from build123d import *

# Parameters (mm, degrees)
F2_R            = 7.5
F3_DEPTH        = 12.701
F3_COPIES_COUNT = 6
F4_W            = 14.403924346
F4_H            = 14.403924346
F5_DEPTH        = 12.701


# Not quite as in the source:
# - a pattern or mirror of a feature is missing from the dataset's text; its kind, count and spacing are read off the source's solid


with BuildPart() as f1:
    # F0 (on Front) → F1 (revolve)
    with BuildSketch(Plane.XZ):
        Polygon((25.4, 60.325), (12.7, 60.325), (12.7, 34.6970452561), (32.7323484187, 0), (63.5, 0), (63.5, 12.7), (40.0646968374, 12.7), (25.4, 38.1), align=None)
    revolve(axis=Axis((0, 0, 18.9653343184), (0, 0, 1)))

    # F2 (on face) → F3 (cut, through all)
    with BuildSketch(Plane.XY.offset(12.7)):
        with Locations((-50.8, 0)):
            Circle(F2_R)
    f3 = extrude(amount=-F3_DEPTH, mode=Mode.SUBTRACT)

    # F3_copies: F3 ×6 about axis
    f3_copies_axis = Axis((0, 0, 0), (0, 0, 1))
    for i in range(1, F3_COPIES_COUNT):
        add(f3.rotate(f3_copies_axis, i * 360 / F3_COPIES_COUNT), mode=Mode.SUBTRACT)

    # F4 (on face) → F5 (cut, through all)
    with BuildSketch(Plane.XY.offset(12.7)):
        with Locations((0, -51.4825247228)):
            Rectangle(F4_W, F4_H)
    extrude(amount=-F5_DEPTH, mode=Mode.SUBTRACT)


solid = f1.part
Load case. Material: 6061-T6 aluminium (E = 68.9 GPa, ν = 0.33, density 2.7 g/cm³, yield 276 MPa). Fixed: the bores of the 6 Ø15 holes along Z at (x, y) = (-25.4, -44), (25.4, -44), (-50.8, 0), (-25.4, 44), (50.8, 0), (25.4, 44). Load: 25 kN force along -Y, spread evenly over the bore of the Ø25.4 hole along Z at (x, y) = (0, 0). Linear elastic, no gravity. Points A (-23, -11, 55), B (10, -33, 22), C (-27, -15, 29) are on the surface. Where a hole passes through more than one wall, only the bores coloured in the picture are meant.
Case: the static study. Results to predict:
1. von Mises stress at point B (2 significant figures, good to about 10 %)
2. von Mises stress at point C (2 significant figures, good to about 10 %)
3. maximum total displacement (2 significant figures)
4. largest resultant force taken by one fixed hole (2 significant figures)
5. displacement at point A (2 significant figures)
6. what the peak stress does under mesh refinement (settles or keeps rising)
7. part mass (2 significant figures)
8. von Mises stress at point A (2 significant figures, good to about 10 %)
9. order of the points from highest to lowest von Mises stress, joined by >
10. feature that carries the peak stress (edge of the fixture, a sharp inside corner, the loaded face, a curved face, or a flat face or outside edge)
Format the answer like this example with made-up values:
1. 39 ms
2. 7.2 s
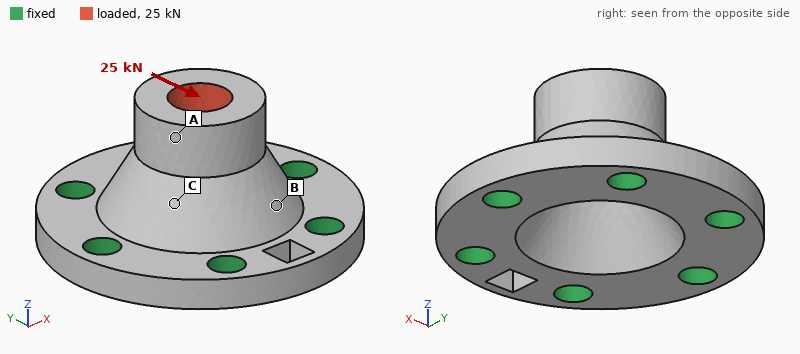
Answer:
1. 36 MPa
2. 22 MPa
3. 54 µm
4. 9.1 kN
5. 42 µm
6. keeps rising
7. 550 g
8. 8.6 MPa
9. B > C > A
10. edge of the fixture
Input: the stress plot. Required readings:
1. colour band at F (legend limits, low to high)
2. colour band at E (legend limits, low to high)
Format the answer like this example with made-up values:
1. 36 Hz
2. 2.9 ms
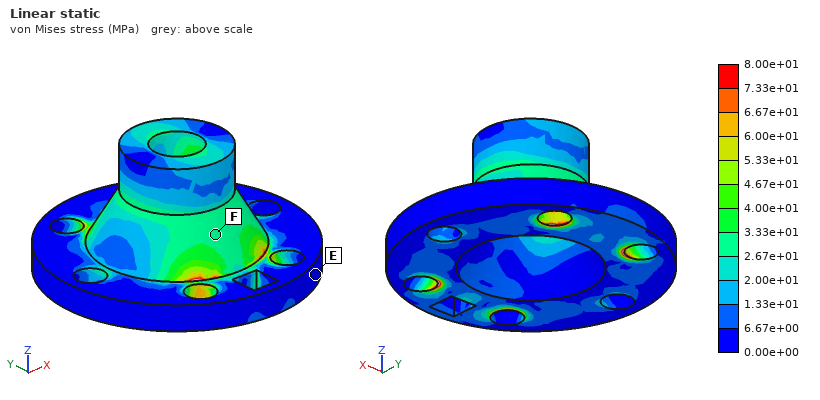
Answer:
1. 2.67e+01 to 3.33e+01 MPa
2. 0.00e+00 to 6.67e+00 MPa
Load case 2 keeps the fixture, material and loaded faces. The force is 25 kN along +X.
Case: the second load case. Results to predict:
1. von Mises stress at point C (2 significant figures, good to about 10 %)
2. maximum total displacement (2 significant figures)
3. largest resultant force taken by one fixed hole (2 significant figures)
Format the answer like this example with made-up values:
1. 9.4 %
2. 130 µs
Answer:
1. 29 MPa
2. 54 µm
3. 10 kN
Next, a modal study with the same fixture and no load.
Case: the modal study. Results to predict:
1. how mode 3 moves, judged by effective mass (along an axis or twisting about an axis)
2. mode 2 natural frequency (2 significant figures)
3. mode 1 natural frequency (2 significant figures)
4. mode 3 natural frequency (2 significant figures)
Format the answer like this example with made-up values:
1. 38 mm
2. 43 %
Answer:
1. along Z
2. 11 kHz
3. 11 kHz
4. 14 kHz
